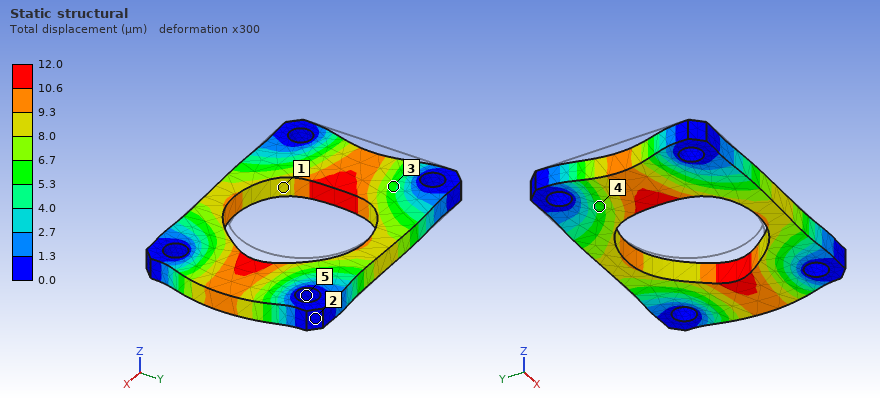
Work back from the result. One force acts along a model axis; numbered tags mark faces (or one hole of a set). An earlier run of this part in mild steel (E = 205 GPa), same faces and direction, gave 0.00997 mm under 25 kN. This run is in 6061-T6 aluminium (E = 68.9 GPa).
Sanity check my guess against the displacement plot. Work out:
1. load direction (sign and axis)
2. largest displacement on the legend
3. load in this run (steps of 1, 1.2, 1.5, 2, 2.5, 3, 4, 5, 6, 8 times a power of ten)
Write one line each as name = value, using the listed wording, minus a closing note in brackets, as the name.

load direction = +X
largest displacement on the legend = 12.0 µm
load in this run = 10 kN
